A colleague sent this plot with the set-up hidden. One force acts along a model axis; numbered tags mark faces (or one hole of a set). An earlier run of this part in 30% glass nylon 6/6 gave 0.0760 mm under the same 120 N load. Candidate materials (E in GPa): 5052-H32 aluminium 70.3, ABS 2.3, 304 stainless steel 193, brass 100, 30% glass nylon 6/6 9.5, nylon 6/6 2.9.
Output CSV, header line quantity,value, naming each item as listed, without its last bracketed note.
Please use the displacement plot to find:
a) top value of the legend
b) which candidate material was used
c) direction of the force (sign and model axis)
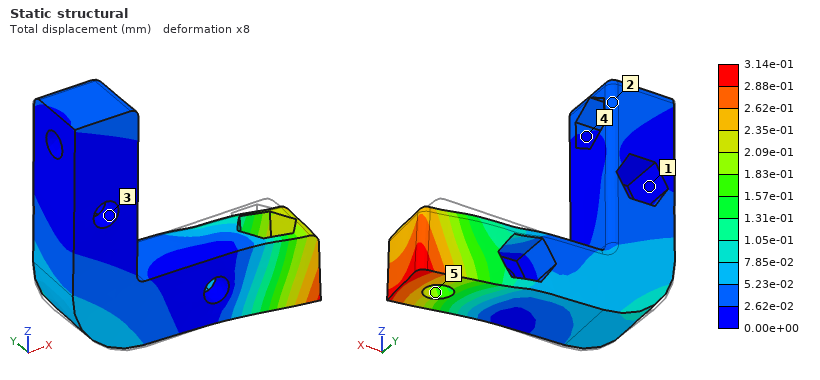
quantity,value
top value of the legend,3.14e-01 mm
which candidate material was used,ABS
direction of the force,-Y
